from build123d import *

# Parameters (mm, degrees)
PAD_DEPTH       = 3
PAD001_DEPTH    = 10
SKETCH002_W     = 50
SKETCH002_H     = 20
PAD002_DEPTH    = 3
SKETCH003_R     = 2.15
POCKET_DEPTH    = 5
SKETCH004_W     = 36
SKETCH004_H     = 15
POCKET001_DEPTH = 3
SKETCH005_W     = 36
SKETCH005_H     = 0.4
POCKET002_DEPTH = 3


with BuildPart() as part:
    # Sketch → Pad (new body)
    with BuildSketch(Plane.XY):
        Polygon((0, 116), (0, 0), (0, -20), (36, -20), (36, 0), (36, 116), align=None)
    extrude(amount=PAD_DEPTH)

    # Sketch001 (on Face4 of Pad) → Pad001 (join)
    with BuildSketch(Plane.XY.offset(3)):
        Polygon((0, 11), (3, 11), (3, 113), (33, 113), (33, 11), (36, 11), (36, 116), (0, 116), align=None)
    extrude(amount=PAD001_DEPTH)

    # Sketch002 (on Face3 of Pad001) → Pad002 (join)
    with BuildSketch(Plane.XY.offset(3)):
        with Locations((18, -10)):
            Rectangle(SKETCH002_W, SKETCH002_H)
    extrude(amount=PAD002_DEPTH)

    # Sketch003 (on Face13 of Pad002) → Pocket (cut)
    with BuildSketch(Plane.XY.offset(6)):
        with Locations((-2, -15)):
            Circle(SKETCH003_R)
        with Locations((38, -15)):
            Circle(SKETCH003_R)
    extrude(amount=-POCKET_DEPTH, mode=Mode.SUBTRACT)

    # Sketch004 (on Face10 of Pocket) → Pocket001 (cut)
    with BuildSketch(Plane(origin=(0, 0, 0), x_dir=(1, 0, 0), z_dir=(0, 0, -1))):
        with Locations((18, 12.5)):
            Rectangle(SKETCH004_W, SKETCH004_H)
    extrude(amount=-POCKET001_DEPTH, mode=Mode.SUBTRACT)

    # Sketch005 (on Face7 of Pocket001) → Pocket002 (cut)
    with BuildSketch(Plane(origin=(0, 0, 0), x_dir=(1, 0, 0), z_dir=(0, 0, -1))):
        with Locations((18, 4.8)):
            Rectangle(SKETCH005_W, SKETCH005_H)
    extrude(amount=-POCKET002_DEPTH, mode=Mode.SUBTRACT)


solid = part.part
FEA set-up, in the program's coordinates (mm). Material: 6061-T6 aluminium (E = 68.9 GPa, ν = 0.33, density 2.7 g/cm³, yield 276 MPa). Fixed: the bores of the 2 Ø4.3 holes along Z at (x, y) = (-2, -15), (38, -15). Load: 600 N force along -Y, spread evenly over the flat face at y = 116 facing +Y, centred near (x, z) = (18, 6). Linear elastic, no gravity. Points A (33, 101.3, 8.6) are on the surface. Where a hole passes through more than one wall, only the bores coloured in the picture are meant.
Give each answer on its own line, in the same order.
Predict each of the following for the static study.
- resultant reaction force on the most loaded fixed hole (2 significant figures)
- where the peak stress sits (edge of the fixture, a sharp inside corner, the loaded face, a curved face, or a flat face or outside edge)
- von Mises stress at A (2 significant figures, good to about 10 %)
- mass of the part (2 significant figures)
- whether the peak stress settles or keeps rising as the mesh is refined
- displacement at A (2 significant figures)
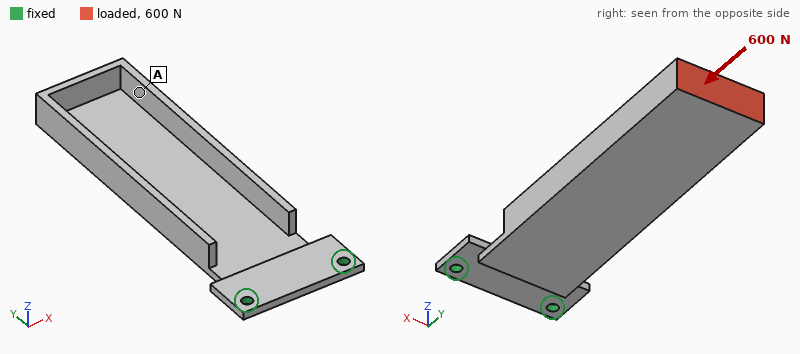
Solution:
330 N
a sharp inside corner
7.7 MPa
62 g
keeps rising
1.1 mm
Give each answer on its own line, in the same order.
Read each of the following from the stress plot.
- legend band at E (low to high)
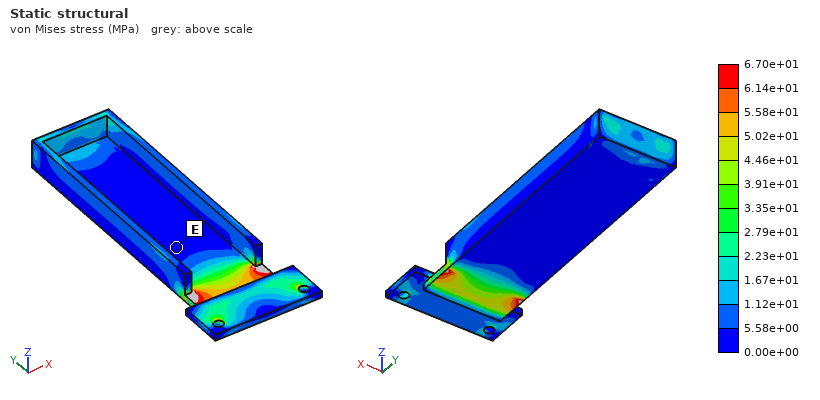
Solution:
0.00e+00 to 5.58e+00 MPa
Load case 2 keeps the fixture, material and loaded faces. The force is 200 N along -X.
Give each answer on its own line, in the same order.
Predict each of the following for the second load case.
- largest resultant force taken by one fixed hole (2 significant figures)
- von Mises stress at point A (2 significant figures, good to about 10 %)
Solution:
670 N
14 MPa
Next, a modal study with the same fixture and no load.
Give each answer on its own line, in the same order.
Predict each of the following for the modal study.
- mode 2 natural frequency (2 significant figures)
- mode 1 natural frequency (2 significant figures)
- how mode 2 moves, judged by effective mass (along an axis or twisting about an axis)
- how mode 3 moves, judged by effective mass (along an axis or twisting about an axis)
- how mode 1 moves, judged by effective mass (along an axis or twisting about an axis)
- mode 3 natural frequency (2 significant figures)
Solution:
770 Hz
140 Hz
along X
along X
along Z
1200 Hz
